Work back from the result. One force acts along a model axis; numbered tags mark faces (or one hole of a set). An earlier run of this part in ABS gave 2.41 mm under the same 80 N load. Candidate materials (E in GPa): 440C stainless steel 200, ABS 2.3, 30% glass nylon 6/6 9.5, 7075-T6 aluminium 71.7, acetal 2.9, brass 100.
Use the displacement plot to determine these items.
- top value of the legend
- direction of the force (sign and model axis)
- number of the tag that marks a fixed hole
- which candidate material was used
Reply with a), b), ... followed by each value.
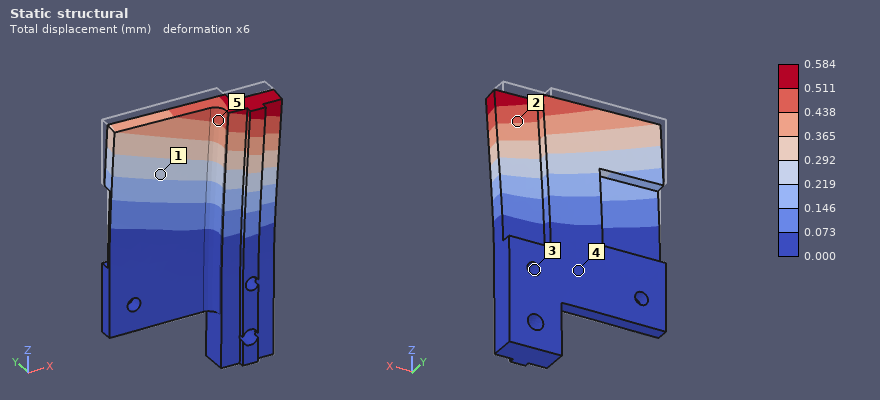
a) 0.584 mm
b) -Y
c) 3
d) 30% glass nylon 6/6
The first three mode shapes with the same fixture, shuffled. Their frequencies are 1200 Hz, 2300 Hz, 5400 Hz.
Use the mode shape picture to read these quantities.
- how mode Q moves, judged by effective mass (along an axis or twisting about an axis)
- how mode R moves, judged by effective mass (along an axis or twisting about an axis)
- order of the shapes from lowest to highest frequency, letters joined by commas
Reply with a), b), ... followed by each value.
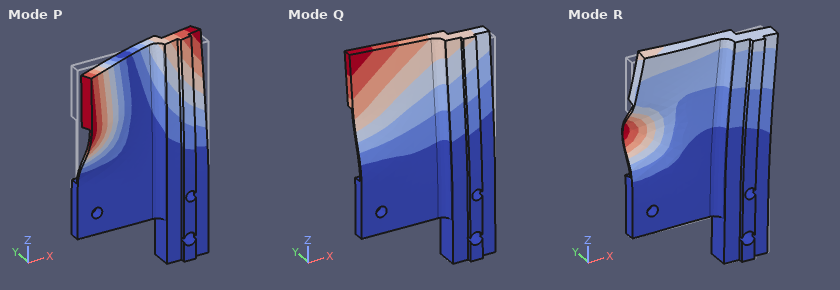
a) along Y
b) along X
c) Q, P, R
